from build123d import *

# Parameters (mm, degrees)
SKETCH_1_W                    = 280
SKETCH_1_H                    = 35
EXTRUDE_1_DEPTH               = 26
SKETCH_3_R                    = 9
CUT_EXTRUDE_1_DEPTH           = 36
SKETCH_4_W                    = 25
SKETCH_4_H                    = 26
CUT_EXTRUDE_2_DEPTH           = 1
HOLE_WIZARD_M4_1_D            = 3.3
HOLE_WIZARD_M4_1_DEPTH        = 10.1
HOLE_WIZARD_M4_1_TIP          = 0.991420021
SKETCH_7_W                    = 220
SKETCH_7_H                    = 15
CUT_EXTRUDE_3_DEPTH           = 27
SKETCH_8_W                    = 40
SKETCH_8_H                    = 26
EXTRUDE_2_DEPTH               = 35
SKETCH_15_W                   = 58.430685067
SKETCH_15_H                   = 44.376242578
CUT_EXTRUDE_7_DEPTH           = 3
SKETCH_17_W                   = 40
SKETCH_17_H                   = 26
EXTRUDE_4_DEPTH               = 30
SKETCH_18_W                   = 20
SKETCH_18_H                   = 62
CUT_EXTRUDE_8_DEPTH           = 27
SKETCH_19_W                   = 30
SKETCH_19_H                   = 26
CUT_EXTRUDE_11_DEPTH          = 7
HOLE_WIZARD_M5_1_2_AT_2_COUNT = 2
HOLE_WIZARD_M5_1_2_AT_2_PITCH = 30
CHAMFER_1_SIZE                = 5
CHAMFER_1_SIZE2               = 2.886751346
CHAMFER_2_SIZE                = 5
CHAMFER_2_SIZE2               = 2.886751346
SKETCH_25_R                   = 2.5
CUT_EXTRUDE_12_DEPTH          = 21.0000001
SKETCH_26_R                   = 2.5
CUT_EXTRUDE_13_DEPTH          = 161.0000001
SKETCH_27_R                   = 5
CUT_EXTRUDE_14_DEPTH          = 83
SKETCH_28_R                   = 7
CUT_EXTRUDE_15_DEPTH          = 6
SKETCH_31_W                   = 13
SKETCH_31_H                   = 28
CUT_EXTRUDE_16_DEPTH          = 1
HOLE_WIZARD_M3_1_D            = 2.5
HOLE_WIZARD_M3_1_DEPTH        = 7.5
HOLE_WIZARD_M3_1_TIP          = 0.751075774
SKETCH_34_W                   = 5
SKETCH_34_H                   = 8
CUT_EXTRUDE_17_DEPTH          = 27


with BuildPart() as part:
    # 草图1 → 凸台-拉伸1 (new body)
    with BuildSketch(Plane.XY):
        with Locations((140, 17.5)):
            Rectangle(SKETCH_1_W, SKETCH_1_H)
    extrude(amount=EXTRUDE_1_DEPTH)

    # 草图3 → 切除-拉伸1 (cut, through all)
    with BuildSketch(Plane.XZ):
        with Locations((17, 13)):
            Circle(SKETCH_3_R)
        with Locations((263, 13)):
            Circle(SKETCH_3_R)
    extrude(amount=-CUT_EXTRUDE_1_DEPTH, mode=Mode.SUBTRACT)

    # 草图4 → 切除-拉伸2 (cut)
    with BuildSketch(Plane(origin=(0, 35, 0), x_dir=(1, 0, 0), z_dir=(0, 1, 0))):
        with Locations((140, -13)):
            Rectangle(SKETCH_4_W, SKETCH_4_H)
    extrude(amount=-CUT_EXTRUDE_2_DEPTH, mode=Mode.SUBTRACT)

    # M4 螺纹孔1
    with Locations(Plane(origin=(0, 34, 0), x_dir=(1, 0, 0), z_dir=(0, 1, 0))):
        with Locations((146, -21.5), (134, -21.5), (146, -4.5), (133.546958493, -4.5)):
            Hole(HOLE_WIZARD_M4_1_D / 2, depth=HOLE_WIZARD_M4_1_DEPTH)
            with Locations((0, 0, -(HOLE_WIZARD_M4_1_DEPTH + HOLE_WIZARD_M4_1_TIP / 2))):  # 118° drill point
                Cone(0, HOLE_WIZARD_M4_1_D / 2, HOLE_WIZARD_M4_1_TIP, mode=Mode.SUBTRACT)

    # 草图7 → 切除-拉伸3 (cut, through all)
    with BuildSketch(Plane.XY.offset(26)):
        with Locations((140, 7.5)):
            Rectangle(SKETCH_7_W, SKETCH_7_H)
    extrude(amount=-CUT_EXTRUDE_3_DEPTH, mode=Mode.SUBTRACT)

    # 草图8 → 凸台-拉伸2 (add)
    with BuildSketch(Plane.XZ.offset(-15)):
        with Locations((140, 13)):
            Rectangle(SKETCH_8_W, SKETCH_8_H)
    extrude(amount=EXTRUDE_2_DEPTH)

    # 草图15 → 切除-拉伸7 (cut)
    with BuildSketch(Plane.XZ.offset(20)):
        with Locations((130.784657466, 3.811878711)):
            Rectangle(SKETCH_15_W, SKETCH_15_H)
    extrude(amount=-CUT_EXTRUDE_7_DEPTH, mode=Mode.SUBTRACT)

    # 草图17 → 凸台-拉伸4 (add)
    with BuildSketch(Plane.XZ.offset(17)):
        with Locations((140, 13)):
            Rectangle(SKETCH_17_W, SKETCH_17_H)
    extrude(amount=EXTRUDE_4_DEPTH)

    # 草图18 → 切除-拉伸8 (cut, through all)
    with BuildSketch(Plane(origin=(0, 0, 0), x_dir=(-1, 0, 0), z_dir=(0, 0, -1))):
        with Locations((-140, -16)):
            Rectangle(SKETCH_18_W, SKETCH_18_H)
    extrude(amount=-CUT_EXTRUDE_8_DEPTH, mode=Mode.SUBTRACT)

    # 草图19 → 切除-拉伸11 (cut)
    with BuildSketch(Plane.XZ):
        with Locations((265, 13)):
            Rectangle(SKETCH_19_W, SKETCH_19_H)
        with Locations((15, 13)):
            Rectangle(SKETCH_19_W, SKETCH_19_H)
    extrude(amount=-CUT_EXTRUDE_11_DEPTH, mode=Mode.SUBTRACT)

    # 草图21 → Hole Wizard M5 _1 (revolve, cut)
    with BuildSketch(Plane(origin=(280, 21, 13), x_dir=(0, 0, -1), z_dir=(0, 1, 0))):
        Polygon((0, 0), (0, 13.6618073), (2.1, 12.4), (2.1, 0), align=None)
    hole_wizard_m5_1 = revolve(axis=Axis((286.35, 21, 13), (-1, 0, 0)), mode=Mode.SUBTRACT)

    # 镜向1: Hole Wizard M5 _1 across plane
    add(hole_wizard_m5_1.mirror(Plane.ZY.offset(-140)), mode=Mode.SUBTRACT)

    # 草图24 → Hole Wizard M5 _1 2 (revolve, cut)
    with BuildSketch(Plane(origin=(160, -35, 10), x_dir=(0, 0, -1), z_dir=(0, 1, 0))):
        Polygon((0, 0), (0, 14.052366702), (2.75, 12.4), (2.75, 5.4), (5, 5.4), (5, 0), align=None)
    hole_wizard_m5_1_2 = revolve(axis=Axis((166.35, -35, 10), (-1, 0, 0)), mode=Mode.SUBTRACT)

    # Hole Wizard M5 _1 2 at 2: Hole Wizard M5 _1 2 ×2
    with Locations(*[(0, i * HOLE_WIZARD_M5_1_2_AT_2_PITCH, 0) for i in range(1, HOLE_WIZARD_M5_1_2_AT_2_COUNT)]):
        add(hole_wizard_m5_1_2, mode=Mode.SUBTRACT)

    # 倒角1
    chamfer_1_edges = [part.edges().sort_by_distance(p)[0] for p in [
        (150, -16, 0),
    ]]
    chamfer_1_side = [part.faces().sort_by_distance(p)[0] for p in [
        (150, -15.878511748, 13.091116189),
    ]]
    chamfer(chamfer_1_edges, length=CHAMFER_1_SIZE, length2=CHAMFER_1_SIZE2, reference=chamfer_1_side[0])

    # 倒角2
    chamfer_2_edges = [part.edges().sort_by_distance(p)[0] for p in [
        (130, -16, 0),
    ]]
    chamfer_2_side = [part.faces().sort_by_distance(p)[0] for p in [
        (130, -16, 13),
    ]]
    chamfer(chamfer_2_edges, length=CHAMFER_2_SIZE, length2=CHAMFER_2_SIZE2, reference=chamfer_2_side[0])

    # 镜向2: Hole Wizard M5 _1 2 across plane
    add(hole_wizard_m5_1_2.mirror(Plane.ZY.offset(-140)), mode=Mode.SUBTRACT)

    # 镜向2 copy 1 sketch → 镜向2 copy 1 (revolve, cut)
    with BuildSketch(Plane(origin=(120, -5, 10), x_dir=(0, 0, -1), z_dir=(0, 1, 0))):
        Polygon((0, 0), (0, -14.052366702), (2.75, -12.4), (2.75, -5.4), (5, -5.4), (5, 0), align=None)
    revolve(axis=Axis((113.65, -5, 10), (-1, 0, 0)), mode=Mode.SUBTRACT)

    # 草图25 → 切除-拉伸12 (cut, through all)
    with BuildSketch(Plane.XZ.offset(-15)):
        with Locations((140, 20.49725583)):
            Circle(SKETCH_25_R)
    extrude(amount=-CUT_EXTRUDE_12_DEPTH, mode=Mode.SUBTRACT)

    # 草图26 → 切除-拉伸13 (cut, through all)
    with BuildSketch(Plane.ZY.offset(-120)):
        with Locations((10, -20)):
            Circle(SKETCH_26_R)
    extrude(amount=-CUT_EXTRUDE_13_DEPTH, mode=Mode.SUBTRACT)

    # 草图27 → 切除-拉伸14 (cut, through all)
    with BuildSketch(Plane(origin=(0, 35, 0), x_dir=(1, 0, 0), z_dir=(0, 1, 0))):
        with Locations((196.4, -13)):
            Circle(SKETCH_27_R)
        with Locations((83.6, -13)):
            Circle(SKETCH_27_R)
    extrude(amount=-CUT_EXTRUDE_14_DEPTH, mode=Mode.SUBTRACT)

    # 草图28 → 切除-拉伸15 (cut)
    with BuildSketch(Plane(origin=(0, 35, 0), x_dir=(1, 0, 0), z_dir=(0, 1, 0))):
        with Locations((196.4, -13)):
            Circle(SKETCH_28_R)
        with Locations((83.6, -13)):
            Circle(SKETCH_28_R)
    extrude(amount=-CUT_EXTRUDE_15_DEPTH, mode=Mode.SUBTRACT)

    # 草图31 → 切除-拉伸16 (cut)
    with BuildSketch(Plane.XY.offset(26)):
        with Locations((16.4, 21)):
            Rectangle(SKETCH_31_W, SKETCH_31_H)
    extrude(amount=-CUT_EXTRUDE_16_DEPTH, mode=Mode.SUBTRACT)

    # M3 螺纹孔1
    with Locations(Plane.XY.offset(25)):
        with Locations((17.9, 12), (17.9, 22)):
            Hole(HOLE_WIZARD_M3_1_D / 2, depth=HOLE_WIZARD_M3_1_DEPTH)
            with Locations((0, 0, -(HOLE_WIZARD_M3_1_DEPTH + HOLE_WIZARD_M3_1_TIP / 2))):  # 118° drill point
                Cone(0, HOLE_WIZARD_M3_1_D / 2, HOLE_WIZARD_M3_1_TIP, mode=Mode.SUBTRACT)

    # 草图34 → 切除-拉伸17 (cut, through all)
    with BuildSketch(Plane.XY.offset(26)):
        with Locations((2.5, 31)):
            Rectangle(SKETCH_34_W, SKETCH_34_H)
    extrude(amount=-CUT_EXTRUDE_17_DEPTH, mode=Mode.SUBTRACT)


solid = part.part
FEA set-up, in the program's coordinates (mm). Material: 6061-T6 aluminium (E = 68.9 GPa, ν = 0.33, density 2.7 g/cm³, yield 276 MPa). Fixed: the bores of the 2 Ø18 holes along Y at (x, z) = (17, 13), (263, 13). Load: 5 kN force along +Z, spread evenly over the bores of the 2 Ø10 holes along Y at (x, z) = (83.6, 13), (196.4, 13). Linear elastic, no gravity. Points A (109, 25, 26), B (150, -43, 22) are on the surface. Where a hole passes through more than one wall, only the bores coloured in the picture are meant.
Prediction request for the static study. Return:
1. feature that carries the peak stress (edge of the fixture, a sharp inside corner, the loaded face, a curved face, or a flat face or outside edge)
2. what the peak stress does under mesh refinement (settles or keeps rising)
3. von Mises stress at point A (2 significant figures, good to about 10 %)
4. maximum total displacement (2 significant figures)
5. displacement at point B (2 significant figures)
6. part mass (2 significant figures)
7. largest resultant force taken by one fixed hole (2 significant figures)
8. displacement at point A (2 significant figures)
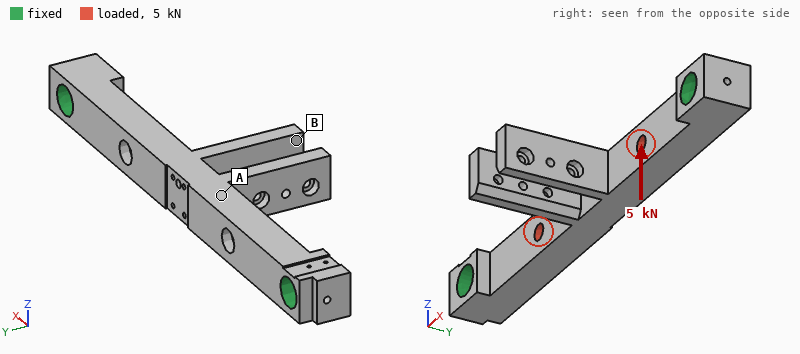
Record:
edge of the fixture
keeps rising
18 MPa
0.15 mm
0.15 mm
450 g
2.5 kN
0.10 mm
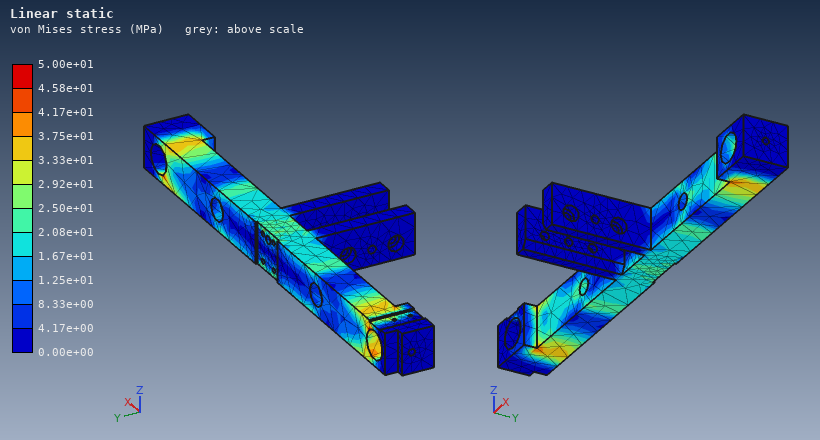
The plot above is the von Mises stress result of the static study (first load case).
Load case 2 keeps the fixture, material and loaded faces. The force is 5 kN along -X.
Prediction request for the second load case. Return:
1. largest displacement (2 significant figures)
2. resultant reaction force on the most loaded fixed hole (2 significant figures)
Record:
5.6 µm
2.5 kN
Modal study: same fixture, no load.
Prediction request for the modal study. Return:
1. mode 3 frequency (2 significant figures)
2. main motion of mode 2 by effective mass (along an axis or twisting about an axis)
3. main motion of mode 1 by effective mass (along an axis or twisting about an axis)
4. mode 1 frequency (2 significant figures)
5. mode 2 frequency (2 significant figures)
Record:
1700 Hz
along Y
along Z
1300 Hz
1500 Hz
